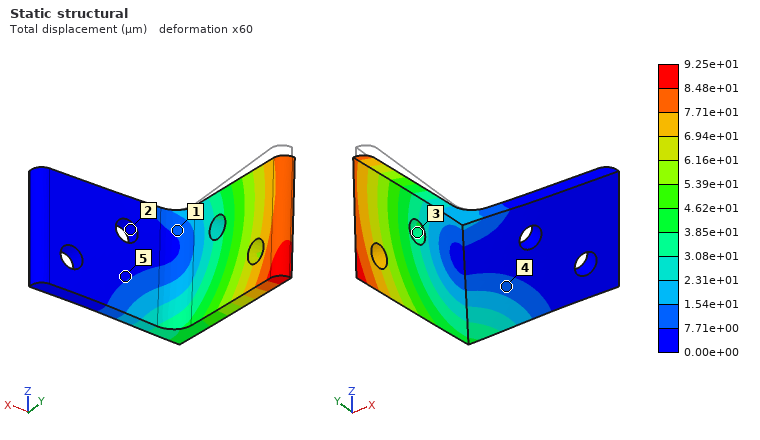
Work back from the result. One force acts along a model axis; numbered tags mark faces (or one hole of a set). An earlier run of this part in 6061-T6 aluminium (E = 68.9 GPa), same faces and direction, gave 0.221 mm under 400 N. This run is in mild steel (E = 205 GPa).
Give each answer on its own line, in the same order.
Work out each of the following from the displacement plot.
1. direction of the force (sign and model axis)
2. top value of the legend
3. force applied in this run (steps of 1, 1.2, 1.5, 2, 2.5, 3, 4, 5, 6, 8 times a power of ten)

-Z
9.25e+01 µm
500 N
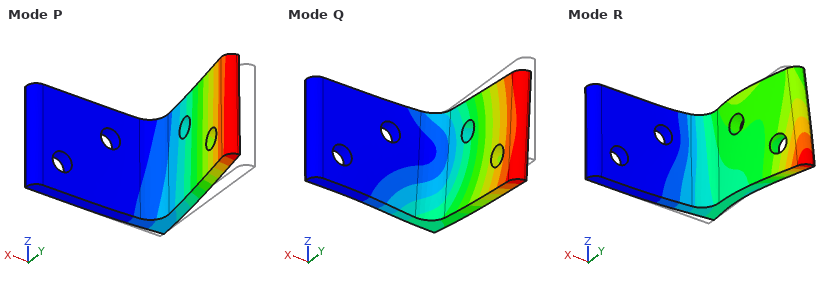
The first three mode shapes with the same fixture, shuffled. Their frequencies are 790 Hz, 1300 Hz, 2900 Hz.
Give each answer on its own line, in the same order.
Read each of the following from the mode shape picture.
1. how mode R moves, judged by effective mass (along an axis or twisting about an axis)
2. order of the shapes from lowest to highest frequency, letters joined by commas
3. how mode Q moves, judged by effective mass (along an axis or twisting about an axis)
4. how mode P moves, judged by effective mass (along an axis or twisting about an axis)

along Y
P, Q, R
along Z
along X
